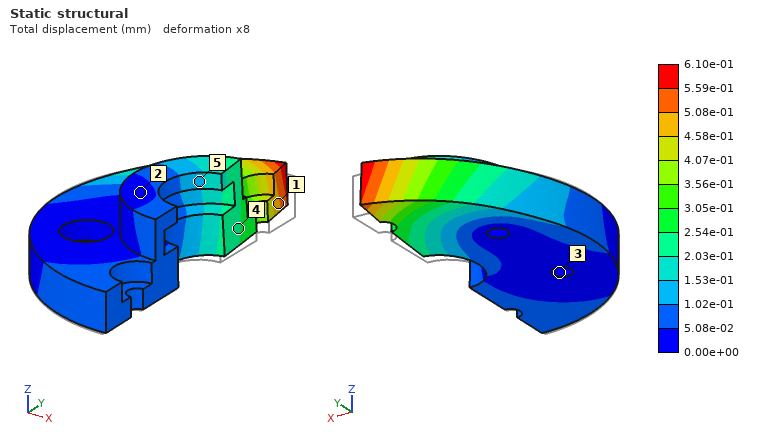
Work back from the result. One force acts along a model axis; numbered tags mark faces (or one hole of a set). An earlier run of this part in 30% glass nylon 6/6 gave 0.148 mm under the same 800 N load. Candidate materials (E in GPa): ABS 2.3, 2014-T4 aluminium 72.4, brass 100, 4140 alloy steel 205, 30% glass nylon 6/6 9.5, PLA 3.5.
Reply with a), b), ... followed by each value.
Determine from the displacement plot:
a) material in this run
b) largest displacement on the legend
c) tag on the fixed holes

a) ABS
b) 6.10e-01 mm
c) 3
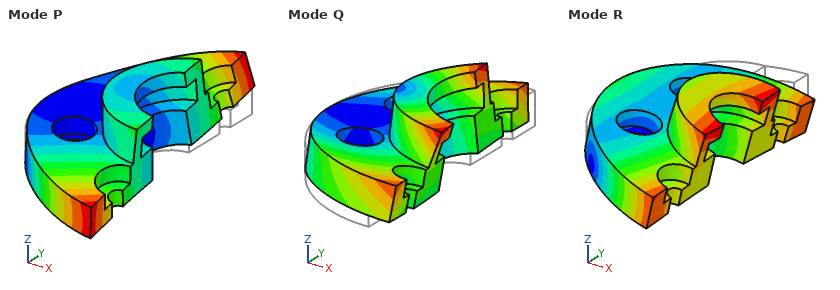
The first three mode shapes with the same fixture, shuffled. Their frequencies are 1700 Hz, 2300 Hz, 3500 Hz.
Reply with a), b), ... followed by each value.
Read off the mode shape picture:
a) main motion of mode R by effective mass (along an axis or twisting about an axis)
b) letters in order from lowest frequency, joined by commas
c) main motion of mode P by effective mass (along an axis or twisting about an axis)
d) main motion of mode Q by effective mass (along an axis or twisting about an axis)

a) along Z
b) R, P, Q
c) twisting about X
d) along Y
